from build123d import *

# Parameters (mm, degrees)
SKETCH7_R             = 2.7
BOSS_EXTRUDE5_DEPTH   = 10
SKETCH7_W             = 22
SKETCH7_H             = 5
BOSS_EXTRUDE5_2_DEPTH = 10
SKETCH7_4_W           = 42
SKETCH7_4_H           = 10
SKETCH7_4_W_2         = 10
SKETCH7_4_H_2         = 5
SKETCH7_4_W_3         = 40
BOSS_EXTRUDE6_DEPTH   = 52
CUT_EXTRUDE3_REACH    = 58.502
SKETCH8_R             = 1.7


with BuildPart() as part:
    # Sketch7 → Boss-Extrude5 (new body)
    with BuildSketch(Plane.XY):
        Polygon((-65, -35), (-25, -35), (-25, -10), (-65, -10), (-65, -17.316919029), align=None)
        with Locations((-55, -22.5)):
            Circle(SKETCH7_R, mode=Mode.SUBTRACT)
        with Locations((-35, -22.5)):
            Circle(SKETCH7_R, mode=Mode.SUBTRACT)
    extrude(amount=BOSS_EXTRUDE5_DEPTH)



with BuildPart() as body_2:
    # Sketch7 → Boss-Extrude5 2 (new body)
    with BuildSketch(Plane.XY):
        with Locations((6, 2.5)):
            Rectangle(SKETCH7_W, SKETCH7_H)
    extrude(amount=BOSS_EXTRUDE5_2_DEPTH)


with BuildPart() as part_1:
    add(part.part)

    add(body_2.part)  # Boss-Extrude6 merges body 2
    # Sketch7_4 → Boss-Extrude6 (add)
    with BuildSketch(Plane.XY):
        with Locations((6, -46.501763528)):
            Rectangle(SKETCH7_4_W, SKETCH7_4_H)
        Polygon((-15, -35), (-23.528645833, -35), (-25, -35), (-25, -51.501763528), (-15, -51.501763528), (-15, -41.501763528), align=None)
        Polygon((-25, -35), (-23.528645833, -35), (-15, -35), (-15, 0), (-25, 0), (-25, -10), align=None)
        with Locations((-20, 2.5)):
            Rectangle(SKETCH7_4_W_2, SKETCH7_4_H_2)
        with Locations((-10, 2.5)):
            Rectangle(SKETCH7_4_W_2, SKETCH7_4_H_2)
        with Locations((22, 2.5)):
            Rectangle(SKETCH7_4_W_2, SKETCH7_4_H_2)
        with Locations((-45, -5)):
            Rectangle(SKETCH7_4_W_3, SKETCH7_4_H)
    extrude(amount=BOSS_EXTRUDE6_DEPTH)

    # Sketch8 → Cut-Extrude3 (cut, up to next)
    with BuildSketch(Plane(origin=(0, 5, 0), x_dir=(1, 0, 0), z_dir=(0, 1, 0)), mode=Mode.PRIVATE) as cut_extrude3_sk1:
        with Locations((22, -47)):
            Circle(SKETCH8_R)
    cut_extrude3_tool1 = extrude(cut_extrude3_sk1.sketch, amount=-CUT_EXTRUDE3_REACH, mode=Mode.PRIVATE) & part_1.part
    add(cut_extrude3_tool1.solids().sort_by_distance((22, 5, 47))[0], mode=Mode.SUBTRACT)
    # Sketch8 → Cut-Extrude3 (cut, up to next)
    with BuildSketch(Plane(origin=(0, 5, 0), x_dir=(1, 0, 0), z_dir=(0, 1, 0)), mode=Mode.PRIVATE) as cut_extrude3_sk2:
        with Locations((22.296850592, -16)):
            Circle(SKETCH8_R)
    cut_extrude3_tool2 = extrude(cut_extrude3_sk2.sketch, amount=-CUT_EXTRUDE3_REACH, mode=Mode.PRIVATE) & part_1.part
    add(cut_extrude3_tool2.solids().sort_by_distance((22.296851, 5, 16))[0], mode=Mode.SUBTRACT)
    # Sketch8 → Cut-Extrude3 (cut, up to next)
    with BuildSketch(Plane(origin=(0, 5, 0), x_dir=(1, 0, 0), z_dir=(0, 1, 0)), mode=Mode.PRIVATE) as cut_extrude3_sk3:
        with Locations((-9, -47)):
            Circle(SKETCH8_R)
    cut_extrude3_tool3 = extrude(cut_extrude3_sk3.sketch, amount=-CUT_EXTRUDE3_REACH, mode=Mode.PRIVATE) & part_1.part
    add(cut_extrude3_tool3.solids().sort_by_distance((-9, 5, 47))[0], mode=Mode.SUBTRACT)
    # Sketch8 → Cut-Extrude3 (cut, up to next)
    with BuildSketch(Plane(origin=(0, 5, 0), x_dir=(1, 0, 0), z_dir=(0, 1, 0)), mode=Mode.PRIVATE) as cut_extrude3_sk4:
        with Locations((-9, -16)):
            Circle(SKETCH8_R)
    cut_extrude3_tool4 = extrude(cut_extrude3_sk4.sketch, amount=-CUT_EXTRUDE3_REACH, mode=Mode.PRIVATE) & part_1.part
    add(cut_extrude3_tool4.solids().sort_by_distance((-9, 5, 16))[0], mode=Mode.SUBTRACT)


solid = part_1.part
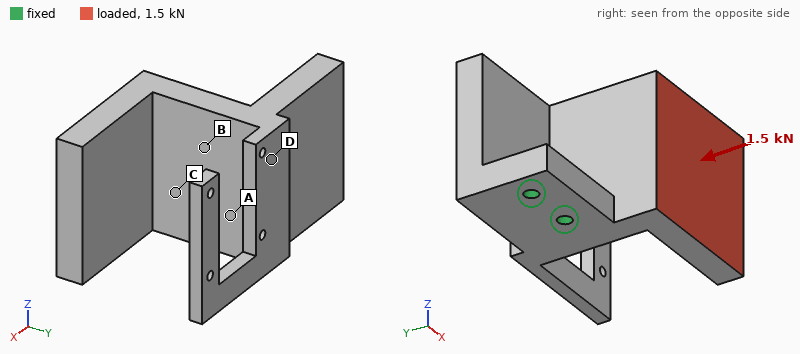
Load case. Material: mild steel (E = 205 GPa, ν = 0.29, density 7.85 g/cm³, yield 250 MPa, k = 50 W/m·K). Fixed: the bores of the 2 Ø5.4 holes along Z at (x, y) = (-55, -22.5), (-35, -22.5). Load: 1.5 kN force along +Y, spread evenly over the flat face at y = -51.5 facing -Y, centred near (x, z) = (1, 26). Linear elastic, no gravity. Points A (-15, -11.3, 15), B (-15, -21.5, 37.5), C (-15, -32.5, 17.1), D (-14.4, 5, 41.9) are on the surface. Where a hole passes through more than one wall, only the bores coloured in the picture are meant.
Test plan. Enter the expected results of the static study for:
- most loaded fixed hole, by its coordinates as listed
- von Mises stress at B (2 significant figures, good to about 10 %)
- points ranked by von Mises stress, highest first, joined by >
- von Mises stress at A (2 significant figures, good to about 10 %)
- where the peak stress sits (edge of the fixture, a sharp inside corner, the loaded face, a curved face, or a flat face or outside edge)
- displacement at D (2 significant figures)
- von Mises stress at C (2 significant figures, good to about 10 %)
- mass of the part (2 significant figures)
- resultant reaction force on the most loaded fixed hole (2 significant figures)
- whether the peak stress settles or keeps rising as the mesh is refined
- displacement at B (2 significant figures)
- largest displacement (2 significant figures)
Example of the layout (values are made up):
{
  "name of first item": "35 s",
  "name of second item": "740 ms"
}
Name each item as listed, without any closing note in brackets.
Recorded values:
{
  "most loaded fixed hole, by its coordinates as listed": "(-35, -22.5)",
  "von Mises stress at B": "21 MPa",
  "points ranked by von Mises stress, highest first, joined by >": "C > B > A > D",
  "von Mises stress at A": "10 MPa",
  "where the peak stress sits": "edge of the fixture",
  "displacement at D": "24 µm",
  "von Mises stress at C": "38 MPa",
  "mass of the part": "690 g",
  "resultant reaction force on the most loaded fixed hole": "3.5 kN",
  "whether the peak stress settles or keeps rising as the mesh is refined": "keeps rising",
  "displacement at B": "21 µm",
  "largest displacement": "94 µm"
}
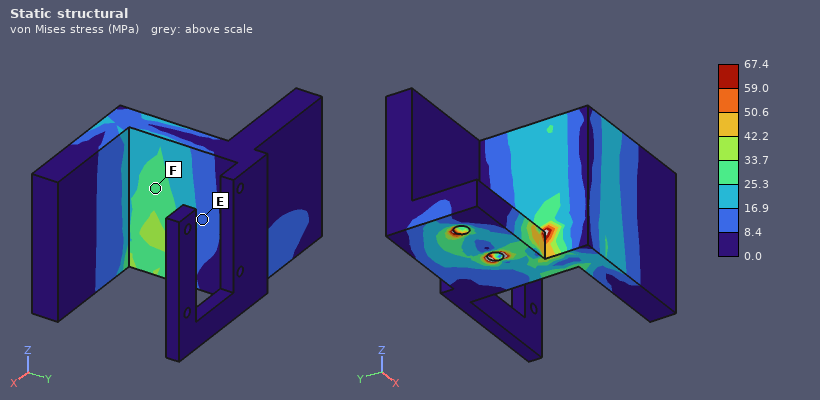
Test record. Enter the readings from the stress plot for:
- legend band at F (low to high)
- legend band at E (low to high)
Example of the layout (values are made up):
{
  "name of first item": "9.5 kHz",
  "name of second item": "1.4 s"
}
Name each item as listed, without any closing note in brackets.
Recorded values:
{
  "legend band at F": "25.3 to 33.7 MPa",
  "legend band at E": "8.4 to 16.9 MPa"
}
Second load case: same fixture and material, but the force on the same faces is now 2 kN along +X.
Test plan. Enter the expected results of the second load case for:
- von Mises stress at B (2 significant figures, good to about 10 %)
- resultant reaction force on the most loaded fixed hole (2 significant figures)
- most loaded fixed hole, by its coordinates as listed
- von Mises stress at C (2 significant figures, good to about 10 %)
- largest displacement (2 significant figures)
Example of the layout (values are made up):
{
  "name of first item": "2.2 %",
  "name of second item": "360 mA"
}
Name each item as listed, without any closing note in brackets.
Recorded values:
{
  "von Mises stress at B": "36 MPa",
  "resultant reaction force on the most loaded fixed hole": "3.1 kN",
  "most loaded fixed hole, by its coordinates as listed": "(-35, -22.5)",
  "von Mises stress at C": "48 MPa",
  "largest displacement": "0.12 mm"
}
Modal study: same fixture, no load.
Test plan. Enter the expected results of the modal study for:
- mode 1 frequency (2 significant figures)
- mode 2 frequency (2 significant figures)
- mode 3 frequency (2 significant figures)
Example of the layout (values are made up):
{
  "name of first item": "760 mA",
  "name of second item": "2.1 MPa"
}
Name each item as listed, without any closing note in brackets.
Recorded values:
{
  "mode 1 frequency": "870 Hz",
  "mode 2 frequency": "1400 Hz",
  "mode 3 frequency": "1600 Hz"
}
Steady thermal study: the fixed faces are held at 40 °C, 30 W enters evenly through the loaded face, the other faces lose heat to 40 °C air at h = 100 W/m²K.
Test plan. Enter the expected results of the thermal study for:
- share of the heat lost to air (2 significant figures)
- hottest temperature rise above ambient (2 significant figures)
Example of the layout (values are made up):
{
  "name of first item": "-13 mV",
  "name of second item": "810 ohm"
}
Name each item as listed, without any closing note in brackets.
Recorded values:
{
  "share of the heat lost to air": "71 %",
  "hottest temperature rise above ambient": "34 K"
}
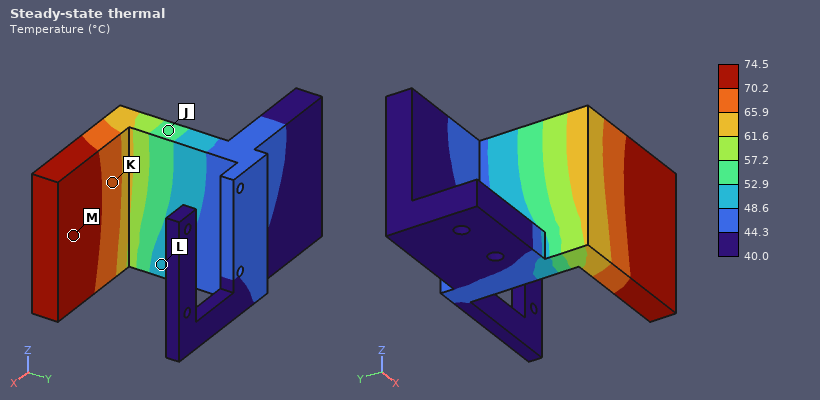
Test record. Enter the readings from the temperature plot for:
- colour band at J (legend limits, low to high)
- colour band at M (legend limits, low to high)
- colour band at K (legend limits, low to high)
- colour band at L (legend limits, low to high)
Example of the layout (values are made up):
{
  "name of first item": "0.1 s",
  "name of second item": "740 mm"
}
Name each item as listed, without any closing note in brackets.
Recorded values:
{
  "colour band at J": "52.9 to 57.2 °C",
  "colour band at M": "70.2 to 74.5 °C",
  "colour band at K": "65.9 to 70.2 °C",
  "colour band at L": "48.6 to 52.9 °C"
}
